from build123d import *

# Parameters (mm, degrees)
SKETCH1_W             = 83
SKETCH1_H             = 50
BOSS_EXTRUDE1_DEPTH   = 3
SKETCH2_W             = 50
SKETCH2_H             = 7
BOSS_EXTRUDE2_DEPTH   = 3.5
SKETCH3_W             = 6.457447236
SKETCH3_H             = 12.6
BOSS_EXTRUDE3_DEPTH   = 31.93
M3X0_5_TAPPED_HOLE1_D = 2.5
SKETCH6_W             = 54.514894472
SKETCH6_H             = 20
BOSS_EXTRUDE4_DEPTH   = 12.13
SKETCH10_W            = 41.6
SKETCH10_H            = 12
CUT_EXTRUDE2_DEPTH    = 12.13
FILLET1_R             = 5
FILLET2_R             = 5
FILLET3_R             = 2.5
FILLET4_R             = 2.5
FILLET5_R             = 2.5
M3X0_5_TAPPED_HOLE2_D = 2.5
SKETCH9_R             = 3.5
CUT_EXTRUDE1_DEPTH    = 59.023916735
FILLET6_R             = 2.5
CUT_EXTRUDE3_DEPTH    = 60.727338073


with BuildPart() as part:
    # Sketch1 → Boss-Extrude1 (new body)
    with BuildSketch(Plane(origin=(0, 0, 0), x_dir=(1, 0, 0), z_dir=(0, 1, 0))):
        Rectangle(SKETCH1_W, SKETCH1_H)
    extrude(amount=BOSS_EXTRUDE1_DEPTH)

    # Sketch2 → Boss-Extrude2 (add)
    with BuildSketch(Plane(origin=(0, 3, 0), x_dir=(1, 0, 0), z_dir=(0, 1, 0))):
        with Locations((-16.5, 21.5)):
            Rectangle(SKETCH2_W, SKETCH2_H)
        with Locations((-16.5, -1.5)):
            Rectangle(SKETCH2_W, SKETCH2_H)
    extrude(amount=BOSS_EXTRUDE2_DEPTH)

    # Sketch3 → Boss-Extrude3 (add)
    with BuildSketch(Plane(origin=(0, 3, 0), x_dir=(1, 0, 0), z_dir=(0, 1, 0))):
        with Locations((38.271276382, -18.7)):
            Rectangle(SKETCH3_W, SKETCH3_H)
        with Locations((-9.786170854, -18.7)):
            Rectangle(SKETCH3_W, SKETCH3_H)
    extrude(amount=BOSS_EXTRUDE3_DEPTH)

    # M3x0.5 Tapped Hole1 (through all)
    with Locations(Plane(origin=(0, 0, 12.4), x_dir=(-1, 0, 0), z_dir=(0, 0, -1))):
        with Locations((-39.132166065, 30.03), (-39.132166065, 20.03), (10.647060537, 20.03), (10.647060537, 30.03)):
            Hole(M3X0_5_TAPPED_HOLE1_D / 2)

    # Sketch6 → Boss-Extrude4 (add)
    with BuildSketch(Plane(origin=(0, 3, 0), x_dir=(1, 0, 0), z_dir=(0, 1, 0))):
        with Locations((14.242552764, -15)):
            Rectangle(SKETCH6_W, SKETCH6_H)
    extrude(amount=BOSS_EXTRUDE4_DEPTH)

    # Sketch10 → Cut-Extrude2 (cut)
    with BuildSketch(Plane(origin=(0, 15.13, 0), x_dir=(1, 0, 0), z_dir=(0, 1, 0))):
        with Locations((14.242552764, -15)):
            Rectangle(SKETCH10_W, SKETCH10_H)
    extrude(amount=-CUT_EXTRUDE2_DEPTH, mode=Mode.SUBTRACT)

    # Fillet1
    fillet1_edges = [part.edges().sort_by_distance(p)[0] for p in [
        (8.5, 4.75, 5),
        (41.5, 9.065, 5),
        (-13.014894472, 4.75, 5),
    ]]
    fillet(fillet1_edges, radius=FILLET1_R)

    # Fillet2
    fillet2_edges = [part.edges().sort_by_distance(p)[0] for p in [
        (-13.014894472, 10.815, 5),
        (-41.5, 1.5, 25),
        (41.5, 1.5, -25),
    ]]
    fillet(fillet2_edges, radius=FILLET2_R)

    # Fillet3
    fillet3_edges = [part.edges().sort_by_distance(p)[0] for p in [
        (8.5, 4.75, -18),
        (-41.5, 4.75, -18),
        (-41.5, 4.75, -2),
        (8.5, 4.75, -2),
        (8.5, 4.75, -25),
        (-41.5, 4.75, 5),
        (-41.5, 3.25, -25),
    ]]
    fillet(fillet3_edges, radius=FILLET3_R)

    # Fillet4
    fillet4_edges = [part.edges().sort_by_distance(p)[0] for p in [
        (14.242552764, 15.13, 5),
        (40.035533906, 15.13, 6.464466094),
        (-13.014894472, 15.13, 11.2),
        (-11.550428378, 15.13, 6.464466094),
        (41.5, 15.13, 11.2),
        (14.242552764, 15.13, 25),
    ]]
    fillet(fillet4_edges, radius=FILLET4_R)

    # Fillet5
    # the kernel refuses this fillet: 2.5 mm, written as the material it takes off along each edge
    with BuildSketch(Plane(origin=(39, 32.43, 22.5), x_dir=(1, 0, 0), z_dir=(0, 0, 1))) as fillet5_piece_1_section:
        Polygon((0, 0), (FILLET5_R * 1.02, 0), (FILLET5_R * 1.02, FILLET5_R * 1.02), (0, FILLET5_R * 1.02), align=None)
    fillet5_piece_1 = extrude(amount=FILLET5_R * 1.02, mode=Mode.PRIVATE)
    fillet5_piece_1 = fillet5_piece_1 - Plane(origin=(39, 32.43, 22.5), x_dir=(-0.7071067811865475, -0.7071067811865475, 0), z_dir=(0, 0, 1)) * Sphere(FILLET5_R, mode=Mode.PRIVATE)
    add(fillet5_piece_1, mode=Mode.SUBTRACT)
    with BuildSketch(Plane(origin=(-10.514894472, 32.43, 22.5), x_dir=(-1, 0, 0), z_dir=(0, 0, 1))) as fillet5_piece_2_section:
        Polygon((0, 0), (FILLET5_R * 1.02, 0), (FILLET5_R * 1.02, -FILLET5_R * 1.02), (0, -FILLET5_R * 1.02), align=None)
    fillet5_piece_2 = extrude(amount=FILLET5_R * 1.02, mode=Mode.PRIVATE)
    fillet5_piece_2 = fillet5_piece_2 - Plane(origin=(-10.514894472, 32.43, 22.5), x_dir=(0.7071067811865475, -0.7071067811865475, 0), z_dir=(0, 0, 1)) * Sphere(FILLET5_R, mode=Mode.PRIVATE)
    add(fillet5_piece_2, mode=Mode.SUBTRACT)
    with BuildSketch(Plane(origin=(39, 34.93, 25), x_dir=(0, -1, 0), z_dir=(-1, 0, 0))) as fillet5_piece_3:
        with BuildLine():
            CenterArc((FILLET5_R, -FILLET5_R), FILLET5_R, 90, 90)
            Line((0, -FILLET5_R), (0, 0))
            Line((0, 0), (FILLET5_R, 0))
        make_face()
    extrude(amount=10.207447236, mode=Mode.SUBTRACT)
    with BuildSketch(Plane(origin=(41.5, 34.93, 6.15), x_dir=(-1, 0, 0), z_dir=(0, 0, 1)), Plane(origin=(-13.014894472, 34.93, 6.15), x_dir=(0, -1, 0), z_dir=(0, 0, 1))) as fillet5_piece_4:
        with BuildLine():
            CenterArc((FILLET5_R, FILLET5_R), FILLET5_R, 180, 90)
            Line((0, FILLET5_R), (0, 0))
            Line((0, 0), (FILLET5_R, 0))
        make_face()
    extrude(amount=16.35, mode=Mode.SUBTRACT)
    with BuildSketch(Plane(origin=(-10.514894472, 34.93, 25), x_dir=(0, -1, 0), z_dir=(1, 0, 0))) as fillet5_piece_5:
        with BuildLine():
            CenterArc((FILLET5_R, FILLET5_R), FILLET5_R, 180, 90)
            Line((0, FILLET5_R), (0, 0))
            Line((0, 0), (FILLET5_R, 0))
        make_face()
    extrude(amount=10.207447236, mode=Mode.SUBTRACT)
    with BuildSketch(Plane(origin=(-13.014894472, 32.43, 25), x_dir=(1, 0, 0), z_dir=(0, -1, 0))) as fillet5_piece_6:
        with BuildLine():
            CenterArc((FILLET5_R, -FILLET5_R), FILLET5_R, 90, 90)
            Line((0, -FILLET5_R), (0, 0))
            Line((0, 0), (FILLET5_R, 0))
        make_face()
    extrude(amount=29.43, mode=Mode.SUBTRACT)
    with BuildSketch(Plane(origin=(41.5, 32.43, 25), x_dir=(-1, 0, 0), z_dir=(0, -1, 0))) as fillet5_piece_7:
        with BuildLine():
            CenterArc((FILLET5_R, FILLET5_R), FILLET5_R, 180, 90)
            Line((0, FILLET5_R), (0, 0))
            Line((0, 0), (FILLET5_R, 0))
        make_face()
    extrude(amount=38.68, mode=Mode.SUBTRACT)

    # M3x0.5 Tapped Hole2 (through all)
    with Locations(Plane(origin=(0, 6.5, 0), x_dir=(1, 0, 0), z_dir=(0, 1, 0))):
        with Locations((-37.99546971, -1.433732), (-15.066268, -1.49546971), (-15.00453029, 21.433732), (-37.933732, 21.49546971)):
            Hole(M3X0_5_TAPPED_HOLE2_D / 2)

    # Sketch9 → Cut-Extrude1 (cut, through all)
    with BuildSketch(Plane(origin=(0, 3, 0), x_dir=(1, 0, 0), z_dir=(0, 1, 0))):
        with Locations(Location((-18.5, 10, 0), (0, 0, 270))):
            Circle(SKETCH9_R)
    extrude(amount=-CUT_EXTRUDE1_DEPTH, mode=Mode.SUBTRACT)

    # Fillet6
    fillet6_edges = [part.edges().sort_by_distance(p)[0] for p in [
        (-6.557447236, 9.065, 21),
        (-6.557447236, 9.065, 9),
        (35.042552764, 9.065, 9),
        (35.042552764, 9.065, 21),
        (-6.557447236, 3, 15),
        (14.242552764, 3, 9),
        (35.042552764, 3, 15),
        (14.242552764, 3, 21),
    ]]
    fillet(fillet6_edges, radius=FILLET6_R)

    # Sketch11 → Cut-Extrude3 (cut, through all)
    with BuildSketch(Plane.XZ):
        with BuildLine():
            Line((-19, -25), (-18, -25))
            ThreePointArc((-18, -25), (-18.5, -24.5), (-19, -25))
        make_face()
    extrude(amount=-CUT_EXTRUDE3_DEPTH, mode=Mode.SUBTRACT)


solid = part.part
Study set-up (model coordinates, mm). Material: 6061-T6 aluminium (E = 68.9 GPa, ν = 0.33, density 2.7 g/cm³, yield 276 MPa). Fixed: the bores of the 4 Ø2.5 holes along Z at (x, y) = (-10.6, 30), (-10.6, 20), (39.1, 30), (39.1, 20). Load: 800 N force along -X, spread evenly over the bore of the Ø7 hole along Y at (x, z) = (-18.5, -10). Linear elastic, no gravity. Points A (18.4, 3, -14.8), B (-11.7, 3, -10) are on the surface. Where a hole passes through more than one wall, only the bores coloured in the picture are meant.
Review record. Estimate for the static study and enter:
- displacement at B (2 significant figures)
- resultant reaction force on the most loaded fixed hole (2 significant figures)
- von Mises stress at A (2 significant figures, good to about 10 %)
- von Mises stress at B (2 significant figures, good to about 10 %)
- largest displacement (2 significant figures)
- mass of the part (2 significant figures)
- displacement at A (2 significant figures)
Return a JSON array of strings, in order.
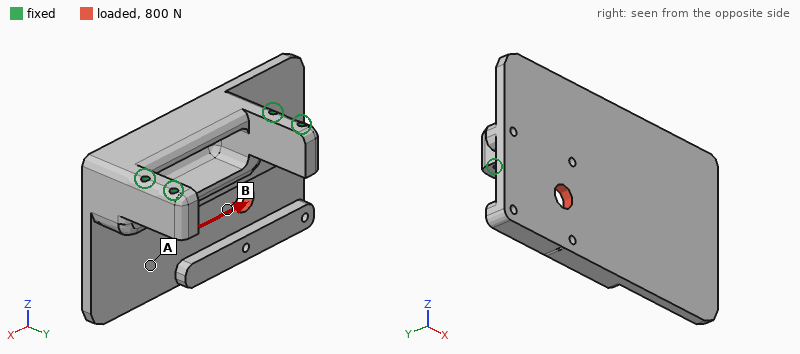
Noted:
["29 µm", "710 N", "5.6 MPa", "12 MPa", "45 µm", "66 g", "24 µm"]
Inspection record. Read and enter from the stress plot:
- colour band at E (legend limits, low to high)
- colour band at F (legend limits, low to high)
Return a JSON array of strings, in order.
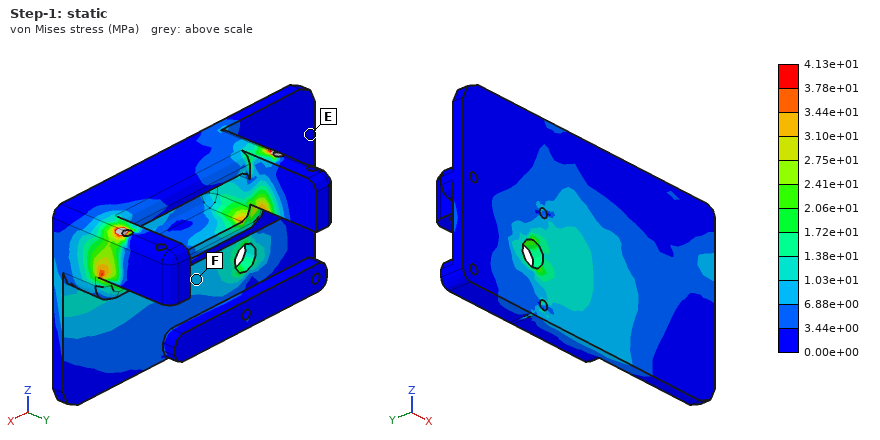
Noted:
["0.00e+00 to 3.44e+00 MPa", "6.88e+00 to 1.03e+01 MPa"]
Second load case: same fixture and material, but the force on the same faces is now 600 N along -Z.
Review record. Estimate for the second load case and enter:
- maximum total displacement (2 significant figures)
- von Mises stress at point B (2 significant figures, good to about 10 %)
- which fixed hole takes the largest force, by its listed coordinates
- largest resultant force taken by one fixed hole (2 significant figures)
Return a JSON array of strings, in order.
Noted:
["73 µm", "8.2 MPa", "(-10.6, 20)", "720 N"]
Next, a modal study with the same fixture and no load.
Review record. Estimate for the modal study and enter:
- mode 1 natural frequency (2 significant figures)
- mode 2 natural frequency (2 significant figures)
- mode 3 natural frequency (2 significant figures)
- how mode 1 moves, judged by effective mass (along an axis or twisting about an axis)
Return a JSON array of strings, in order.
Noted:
["1900 Hz", "2800 Hz", "4100 Hz", "along Y"]
